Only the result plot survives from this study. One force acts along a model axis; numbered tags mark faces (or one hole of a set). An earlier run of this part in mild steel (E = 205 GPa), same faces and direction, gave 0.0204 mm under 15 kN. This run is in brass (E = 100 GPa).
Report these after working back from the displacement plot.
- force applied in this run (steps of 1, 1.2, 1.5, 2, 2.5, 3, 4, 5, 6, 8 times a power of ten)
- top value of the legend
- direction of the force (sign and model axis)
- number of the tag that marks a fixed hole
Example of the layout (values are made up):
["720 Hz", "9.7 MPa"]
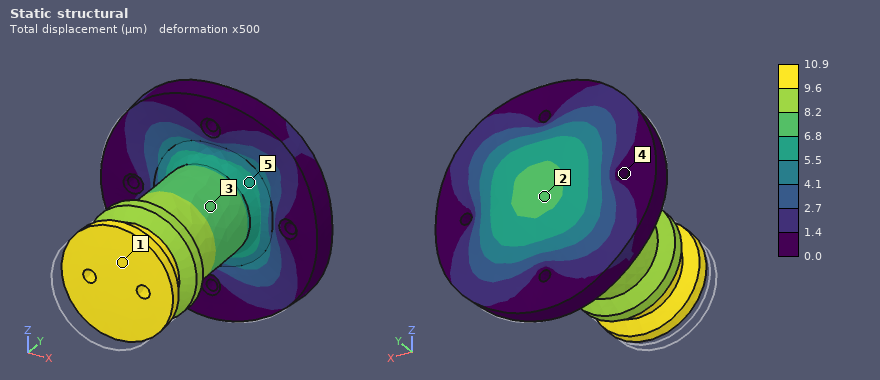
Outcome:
["4 kN", "10.9 µm", "+Y", "4"]
